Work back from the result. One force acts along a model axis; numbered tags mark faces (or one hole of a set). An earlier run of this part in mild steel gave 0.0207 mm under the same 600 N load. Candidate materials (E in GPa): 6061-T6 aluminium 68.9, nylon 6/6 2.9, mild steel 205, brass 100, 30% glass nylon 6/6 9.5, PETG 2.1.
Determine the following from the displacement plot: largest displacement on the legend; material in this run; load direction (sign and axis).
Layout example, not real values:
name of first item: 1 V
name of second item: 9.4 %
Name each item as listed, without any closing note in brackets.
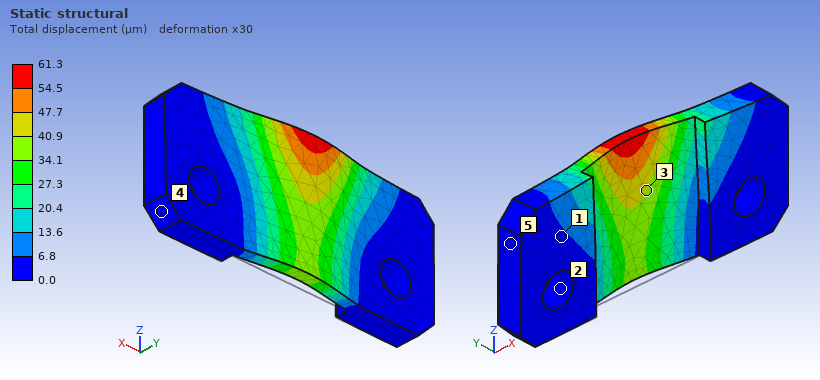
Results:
largest displacement on the legend: 61.3 µm
material in this run: 6061-T6 aluminium
load direction: +Y
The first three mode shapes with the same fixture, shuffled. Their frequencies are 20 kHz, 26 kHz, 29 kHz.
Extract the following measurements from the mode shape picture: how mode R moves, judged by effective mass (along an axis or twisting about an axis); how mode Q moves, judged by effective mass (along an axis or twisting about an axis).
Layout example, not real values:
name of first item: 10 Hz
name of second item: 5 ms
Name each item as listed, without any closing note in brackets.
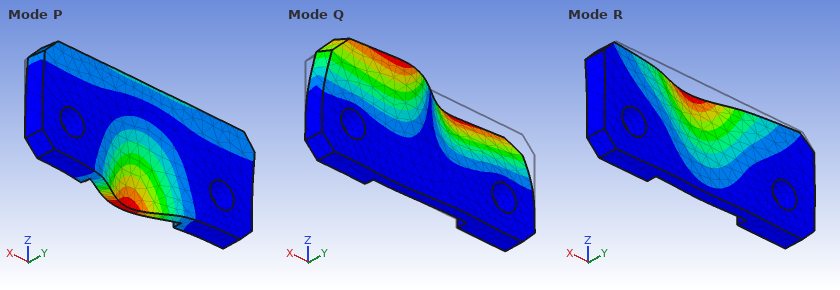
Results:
how mode R moves, judged by effective mass: along Y
how mode Q moves, judged by effective mass: twisting about Z
